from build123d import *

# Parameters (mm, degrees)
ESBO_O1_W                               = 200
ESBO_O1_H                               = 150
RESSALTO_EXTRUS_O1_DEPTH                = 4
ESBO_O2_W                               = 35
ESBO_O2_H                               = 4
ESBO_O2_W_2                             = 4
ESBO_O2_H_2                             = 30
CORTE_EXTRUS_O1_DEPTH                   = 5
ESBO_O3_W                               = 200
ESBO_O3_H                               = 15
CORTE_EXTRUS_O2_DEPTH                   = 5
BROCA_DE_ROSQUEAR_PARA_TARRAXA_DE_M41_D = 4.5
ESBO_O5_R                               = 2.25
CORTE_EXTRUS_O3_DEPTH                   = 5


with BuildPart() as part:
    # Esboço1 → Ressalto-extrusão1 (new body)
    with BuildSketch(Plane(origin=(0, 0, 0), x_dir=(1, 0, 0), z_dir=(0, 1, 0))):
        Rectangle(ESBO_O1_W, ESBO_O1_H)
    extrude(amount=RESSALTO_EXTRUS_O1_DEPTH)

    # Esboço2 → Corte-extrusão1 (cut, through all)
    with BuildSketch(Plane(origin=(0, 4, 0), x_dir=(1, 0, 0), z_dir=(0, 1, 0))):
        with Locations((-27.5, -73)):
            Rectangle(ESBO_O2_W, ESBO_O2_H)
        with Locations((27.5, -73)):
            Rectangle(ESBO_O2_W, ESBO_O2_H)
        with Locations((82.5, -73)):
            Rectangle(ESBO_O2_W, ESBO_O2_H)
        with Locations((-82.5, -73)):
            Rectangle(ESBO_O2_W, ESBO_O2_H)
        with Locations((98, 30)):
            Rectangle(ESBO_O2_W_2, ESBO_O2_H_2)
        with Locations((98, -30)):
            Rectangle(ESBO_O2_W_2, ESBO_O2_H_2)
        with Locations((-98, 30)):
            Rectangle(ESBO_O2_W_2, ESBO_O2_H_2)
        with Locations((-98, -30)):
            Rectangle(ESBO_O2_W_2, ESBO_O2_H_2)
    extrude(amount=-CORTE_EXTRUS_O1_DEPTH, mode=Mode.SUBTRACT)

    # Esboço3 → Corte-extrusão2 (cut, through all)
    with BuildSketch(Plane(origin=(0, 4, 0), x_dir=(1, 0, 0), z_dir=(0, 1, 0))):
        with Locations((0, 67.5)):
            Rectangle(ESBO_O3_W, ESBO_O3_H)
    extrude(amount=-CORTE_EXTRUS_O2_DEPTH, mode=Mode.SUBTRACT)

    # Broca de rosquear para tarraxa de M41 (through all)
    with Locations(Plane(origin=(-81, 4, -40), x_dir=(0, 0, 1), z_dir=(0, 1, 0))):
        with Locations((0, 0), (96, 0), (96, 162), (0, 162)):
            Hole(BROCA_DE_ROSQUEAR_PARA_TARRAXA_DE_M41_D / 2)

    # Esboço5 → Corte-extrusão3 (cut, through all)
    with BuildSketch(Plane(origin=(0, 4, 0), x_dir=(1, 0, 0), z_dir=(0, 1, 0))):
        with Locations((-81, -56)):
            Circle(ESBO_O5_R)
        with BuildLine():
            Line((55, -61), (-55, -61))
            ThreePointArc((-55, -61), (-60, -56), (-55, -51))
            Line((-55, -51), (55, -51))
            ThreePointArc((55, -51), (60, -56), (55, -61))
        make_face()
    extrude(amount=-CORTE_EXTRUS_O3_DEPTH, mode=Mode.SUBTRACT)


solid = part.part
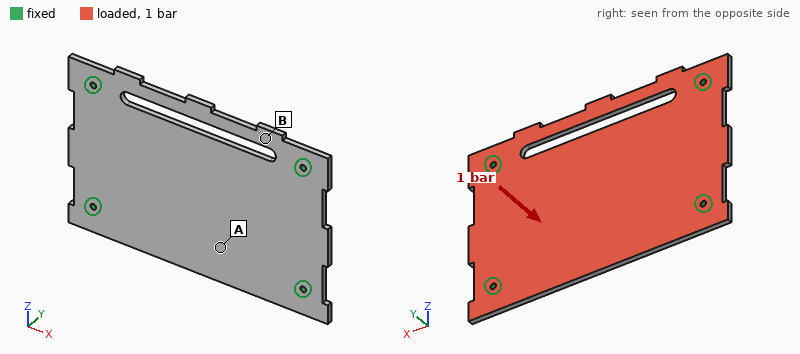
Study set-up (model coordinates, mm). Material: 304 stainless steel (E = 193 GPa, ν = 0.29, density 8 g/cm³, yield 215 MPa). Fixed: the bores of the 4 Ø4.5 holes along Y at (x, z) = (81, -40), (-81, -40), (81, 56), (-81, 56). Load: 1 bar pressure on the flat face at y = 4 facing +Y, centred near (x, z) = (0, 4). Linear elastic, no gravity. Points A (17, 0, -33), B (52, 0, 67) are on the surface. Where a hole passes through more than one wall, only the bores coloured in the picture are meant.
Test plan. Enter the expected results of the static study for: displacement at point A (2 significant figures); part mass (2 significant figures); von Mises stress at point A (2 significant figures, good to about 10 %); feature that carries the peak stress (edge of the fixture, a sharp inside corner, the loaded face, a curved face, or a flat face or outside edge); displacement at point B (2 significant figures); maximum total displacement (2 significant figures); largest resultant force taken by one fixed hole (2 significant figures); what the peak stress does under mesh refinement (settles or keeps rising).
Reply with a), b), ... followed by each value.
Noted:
a) 0.22 mm
b) 790 g
c) 41 MPa
d) edge of the fixture
e) 0.068 mm
f) 0.25 mm
g) 660 N
h) keeps rising
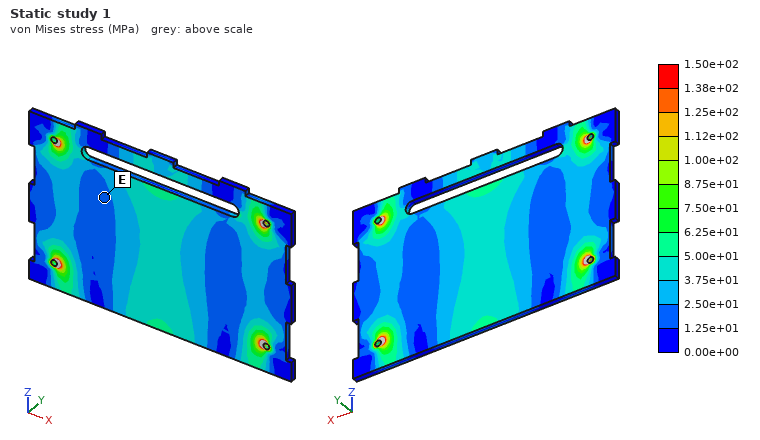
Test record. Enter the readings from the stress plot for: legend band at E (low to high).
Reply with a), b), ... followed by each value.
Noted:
a) 1.25e+01 to 2.50e+01 MPa
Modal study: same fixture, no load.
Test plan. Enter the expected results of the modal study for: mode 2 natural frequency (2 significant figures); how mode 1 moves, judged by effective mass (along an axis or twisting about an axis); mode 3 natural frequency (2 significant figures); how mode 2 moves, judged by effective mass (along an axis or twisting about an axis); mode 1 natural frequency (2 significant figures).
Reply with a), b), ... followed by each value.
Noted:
a) 910 Hz
b) along Y
c) 1100 Hz
d) twisting about X
e) 650 Hz
